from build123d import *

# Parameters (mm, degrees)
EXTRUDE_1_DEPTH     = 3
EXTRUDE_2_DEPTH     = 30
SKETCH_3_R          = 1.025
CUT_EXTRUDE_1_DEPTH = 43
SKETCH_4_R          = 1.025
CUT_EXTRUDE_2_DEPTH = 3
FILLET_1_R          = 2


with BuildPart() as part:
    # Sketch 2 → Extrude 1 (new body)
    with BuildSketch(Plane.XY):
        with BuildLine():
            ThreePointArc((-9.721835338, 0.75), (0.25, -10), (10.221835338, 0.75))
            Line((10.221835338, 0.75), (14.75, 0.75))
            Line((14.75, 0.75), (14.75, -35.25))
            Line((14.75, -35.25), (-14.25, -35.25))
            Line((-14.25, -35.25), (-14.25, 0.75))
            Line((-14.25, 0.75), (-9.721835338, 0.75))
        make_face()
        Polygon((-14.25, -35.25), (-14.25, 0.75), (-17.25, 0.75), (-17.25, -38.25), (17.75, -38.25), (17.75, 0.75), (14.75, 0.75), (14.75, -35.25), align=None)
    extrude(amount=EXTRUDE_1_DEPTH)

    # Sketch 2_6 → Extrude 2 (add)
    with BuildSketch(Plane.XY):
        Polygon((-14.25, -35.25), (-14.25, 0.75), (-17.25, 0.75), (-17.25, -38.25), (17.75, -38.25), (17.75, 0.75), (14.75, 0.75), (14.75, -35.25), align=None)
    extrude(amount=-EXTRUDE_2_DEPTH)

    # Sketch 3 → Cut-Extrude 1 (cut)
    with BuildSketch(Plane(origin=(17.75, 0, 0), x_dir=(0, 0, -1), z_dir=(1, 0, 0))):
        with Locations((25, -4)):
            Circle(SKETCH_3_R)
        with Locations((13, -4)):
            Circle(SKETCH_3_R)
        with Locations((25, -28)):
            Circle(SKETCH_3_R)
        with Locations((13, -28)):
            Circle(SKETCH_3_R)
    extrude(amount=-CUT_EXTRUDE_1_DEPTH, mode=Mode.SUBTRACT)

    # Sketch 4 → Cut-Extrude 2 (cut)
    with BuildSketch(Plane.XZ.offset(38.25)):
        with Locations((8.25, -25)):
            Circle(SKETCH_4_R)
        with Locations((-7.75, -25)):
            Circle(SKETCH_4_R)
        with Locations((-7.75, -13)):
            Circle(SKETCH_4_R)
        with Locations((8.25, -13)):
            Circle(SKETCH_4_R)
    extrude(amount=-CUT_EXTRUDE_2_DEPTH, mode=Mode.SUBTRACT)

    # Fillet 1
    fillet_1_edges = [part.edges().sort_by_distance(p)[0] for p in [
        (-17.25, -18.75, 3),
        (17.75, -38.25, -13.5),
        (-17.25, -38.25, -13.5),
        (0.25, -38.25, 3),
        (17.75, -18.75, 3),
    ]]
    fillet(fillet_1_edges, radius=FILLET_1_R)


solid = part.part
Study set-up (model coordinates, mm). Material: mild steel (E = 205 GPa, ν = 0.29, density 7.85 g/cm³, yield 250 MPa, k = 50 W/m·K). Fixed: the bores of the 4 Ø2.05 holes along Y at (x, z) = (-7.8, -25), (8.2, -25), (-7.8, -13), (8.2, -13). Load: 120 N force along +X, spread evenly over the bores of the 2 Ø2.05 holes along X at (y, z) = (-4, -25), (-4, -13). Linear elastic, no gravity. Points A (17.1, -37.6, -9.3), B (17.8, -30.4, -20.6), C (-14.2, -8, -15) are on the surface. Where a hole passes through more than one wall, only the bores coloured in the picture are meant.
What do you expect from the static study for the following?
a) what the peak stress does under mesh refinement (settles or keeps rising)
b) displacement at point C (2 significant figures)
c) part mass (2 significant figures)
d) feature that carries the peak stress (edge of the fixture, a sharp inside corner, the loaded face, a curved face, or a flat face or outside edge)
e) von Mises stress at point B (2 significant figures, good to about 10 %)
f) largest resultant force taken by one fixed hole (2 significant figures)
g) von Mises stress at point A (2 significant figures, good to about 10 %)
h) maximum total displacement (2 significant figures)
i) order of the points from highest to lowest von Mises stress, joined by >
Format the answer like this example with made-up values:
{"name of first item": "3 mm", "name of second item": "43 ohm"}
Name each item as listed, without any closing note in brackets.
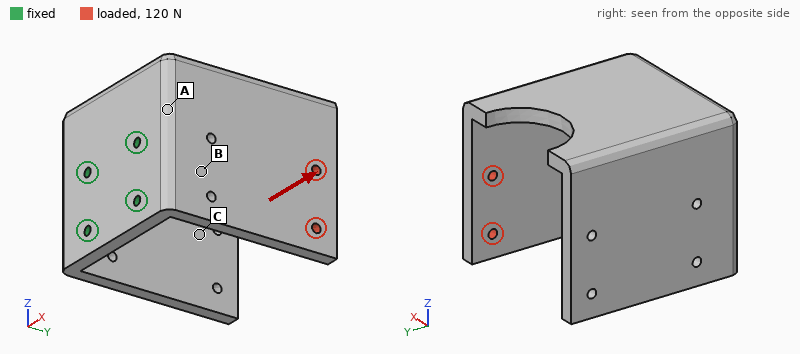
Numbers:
{"what the peak stress does under mesh refinement": "keeps rising", "displacement at point C": "16 µm", "part mass": "100 g", "feature that carries the peak stress": "edge of the fixture", "von Mises stress at point B": "26 MPa", "largest resultant force taken by one fixed hole": "220 N", "von Mises stress at point A": "7.0 MPa", "maximum total displacement": "79 µm", "order of the points from highest to lowest von Mises stress, joined by >": "B > A > C"}
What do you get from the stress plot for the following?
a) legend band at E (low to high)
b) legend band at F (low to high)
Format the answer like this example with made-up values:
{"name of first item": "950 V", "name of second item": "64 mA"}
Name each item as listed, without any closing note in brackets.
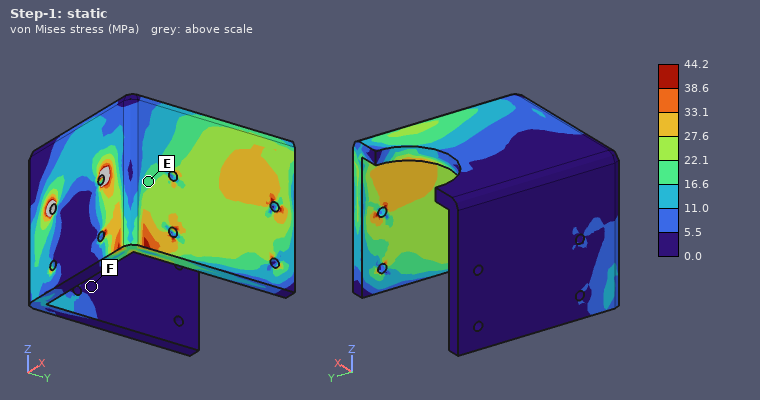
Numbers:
{"legend band at E": "16.6 to 22.1 MPa", "legend band at F": "0.0 to 5.5 MPa"}
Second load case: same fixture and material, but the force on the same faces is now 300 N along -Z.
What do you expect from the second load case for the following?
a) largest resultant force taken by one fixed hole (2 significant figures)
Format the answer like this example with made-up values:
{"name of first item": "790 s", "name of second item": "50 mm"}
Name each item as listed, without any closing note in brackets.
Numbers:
{"largest resultant force taken by one fixed hole": "550 N"}
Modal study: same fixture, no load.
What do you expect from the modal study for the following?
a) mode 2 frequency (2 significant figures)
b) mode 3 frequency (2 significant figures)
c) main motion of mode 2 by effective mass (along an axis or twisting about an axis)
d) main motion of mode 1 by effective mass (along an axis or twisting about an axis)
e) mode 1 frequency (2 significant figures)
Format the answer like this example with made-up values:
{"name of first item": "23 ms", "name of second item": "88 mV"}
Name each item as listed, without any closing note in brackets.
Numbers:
{"mode 2 frequency": "2600 Hz", "mode 3 frequency": "3200 Hz", "main motion of mode 2 by effective mass": "along Z", "main motion of mode 1 by effective mass": "along X", "mode 1 frequency": "1900 Hz"}
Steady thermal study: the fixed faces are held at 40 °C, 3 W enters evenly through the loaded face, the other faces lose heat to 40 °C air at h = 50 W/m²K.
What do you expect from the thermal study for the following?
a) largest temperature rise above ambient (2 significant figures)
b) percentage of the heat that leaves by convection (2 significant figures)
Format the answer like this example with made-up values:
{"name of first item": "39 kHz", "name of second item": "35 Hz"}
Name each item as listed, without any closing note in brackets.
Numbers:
{"largest temperature rise above ambient": "19 K", "percentage of the heat that leaves by convection": "52 %"}
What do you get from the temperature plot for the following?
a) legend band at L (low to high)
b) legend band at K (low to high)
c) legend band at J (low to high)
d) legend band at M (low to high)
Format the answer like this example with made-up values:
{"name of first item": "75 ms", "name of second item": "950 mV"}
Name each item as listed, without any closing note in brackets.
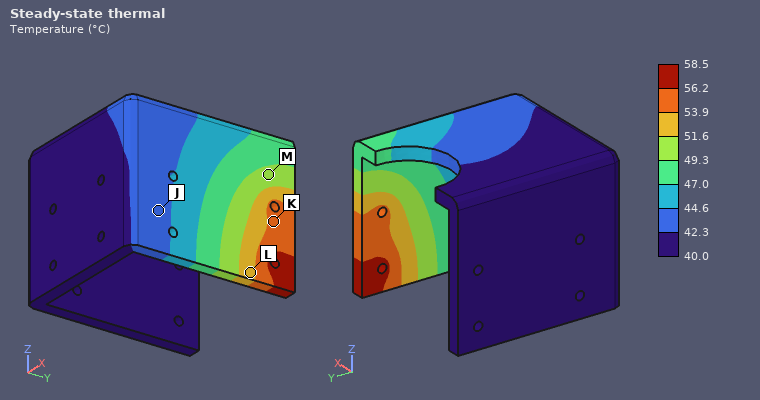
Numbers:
{"legend band at L": "51.6 to 53.9 °C", "legend band at K": "53.9 to 56.2 °C", "legend band at J": "42.3 to 44.6 °C", "legend band at M": "49.3 to 51.6 °C"}
